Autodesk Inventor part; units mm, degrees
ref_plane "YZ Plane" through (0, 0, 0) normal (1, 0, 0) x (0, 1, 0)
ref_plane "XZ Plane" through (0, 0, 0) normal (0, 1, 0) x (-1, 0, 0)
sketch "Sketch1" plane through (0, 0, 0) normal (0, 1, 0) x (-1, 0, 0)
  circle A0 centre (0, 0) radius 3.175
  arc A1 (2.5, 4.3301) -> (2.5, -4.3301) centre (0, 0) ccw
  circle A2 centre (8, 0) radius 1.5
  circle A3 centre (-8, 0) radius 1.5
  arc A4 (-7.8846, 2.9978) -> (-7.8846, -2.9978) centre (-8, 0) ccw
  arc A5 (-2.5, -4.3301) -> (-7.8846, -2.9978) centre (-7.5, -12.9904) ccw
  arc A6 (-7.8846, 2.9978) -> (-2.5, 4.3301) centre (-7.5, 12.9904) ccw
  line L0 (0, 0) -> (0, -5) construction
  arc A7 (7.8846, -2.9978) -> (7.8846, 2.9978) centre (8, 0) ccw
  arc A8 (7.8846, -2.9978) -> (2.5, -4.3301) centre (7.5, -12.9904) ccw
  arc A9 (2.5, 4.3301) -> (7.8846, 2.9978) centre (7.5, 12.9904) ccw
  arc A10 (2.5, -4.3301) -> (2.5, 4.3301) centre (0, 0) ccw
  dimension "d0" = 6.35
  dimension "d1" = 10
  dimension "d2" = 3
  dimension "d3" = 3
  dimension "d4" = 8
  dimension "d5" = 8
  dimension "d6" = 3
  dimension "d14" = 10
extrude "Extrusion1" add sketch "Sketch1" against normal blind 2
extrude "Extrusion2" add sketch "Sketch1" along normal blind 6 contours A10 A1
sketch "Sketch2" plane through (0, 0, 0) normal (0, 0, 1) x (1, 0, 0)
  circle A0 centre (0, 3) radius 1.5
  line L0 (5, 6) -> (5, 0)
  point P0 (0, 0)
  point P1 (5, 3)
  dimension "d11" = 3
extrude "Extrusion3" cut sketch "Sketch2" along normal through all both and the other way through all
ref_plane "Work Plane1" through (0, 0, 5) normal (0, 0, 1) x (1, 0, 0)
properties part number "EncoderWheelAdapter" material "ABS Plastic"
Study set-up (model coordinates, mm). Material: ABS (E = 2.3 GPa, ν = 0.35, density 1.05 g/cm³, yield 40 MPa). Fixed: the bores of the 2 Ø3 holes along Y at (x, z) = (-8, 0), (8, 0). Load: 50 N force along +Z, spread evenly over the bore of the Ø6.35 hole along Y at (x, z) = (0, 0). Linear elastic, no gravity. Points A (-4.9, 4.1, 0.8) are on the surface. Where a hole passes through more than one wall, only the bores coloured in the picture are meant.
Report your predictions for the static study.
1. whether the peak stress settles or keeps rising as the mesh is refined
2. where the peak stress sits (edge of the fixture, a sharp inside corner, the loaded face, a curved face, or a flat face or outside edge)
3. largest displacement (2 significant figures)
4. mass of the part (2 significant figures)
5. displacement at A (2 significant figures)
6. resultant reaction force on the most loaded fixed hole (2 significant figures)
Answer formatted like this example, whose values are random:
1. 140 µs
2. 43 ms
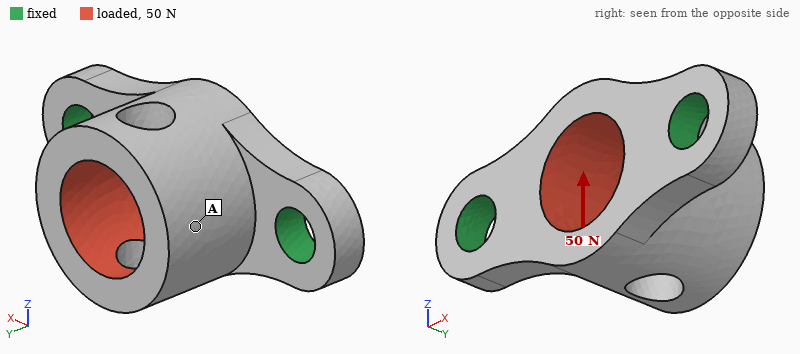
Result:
1. keeps rising
2. edge of the fixture
3. 0.13 mm
4. 0.49 g
5. 0.083 mm
6. 25 N
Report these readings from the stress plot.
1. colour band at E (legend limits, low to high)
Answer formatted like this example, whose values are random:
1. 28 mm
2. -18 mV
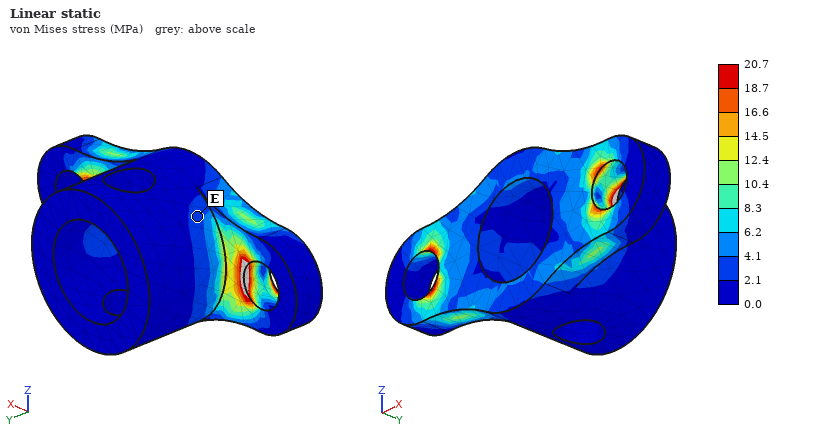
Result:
1. 2.1 to 4.1 MPa
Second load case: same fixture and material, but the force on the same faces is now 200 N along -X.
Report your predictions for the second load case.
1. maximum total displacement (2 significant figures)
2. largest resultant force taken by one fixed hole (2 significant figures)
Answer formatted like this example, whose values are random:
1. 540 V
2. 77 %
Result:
1. 89 µm
2. 110 N
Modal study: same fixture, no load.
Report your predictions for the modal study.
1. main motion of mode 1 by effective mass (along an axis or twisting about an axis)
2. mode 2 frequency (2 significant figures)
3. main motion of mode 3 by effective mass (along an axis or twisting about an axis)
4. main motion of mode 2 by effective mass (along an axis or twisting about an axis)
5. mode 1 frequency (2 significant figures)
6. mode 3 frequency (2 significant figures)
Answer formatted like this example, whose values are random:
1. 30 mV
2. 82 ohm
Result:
1. along Z
2. 12 kHz
3. along X
4. along Y
5. 5500 Hz
6. 14 kHz
